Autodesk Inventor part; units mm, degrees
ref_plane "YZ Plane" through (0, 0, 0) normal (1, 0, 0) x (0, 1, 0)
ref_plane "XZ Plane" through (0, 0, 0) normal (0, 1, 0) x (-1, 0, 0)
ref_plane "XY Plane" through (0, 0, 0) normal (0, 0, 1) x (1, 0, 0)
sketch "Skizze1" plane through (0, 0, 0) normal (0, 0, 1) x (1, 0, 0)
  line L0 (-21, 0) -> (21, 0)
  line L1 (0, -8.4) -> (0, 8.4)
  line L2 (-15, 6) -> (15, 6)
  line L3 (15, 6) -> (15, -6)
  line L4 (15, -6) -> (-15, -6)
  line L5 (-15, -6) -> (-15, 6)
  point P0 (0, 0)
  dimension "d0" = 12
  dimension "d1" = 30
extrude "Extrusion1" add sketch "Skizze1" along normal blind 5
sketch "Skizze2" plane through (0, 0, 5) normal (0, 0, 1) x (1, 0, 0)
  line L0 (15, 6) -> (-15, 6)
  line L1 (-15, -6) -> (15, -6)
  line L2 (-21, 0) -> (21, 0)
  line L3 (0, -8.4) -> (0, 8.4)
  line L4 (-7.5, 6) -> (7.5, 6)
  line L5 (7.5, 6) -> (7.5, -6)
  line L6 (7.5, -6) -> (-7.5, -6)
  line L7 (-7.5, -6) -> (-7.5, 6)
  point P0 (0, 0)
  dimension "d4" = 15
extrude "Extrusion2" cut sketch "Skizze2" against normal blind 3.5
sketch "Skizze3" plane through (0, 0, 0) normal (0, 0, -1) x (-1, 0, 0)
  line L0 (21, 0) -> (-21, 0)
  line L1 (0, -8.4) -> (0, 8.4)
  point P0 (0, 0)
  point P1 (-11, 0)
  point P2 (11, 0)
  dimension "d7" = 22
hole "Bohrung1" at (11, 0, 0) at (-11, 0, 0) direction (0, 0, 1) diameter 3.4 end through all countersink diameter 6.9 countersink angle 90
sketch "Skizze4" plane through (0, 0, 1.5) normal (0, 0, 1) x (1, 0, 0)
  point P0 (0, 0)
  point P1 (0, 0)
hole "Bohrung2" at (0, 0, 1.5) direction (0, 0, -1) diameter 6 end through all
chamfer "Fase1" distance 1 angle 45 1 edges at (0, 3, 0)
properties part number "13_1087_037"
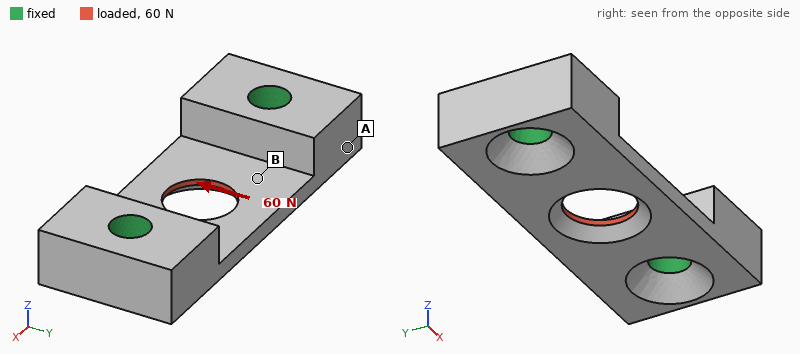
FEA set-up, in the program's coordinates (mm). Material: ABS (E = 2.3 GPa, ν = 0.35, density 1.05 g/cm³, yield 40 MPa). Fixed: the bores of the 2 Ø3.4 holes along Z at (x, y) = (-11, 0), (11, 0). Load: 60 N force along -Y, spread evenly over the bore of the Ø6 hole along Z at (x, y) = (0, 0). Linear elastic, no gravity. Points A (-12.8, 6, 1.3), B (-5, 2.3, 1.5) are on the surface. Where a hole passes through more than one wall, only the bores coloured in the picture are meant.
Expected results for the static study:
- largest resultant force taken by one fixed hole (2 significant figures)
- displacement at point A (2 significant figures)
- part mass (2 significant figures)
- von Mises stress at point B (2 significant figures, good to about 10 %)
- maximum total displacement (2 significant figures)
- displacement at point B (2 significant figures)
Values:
30 N
7.1 µm
1.0 g
4.7 MPa
39 µm
19 µm
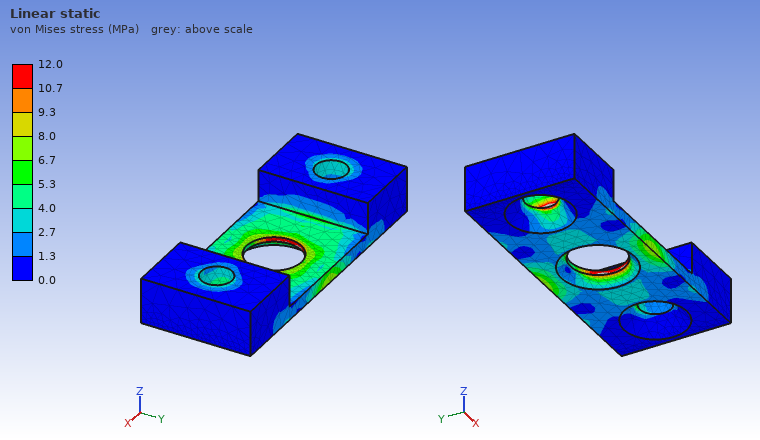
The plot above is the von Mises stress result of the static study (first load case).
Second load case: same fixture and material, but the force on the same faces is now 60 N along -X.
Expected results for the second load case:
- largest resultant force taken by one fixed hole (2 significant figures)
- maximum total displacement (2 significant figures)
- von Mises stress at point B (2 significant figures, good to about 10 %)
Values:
30 N
15 µm
4.0 MPa
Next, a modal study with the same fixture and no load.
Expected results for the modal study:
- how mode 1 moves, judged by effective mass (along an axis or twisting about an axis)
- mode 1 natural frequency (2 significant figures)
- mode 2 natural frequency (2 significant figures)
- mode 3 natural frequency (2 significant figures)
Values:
along Z
8100 Hz
9300 Hz
16 kHz
